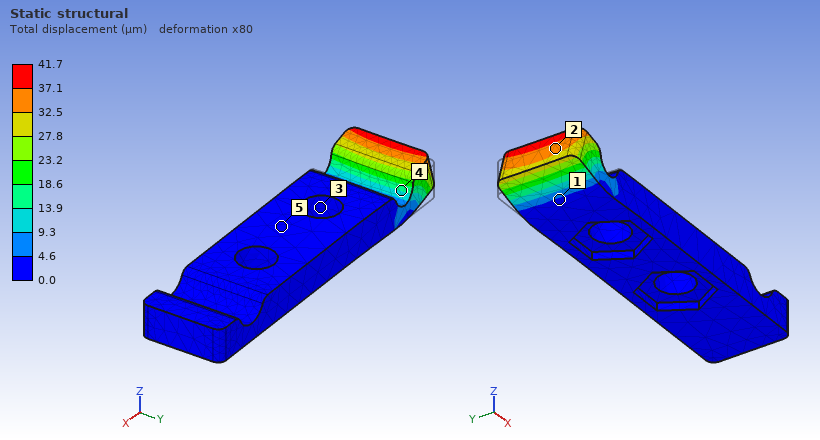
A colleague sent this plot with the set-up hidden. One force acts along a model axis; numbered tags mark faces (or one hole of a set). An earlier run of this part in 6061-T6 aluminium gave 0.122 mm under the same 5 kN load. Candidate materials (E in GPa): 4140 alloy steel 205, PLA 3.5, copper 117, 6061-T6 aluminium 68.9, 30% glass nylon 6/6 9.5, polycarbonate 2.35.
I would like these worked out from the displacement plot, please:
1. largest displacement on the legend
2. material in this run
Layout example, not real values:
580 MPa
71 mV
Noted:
41.7 µm
4140 alloy steel
